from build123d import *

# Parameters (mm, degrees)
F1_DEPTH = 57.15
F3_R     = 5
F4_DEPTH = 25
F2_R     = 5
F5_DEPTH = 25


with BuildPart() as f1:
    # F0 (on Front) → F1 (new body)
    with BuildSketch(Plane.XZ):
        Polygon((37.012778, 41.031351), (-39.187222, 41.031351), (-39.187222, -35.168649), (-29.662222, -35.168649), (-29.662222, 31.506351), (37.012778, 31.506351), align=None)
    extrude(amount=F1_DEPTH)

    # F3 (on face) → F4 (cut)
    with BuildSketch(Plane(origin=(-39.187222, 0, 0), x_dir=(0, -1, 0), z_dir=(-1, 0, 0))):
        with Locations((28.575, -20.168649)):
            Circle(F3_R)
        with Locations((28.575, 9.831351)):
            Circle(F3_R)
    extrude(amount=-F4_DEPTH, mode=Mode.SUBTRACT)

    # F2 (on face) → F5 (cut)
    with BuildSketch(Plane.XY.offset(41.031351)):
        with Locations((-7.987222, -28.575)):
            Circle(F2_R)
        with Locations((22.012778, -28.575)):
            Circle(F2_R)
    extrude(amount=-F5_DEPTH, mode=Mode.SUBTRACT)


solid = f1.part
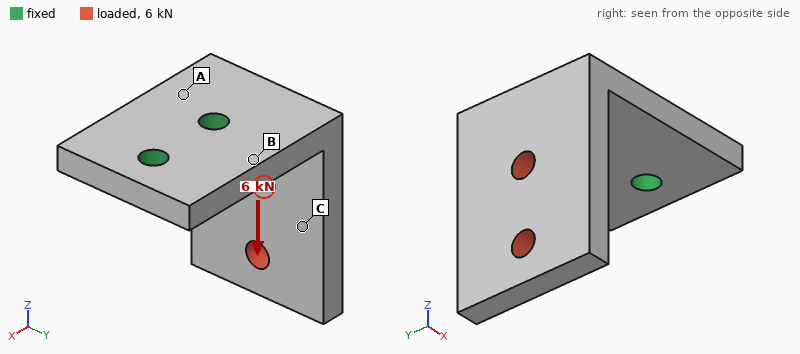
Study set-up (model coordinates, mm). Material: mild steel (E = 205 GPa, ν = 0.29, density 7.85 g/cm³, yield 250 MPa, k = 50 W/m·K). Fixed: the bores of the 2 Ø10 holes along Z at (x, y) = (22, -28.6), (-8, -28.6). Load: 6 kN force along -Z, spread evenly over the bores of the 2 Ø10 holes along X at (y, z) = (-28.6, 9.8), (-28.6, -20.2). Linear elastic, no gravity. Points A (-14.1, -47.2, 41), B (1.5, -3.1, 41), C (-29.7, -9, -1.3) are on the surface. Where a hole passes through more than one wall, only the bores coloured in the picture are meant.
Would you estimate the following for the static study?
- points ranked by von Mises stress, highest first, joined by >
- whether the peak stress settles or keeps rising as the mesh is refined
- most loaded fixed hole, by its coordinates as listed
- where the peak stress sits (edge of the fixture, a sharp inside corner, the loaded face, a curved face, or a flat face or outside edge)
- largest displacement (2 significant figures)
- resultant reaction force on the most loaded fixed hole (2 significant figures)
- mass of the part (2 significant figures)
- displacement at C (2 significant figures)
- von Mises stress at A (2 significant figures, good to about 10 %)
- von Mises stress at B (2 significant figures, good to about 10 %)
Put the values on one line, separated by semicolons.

A > B > C; keeps rising; (-8, -28.6); edge of the fixture; 0.19 mm; 7.5 kN; 590 g; 0.10 mm; 84 MPa; 41 MPa
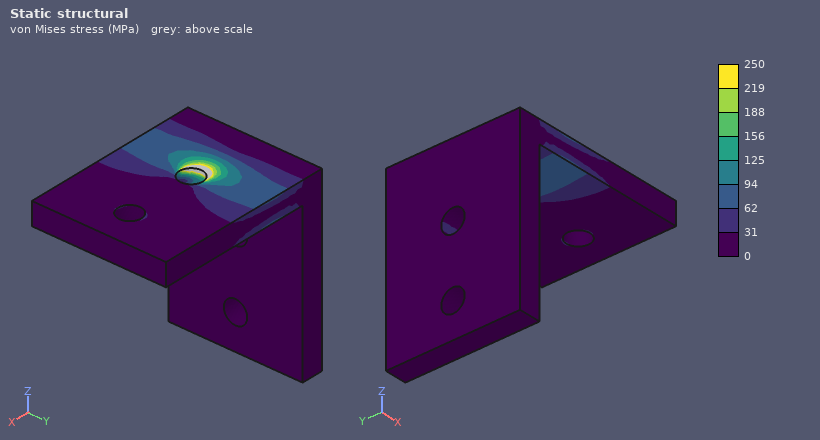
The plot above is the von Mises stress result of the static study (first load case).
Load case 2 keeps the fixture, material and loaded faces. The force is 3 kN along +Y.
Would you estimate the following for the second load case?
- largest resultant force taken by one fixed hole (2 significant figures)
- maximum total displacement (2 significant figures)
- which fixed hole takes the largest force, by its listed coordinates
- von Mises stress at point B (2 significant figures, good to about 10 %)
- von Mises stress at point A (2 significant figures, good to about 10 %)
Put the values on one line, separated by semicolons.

4.7 kN; 0.18 mm; (-8, -28.6); 52 MPa; 60 MPa
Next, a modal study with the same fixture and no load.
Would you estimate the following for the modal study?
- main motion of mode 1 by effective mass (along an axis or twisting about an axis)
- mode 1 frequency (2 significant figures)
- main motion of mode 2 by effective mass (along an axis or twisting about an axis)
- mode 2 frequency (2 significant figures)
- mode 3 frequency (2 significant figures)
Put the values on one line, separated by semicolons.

along X; 1000 Hz; along Y; 1500 Hz; 3700 Hz
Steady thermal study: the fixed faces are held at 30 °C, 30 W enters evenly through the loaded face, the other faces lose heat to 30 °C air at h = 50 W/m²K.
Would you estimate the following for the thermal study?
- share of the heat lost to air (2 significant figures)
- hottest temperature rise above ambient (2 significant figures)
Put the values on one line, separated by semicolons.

55 %; 44 K
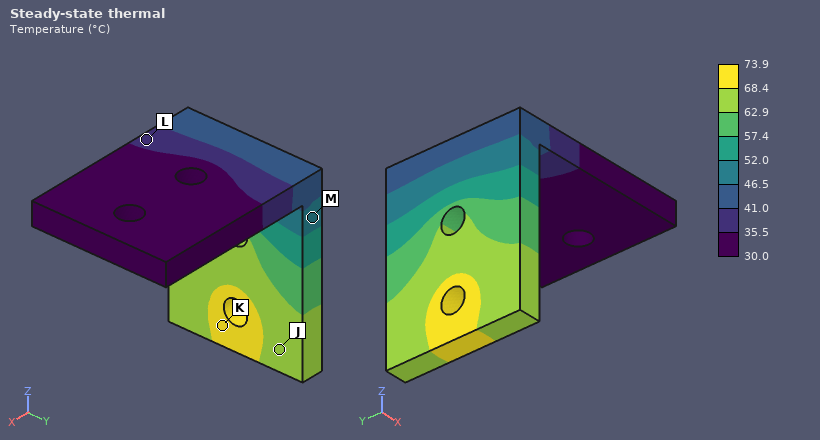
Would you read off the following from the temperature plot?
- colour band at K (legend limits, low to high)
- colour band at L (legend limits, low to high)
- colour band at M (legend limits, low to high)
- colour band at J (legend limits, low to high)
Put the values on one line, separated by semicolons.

68.4 to 73.9 °C; 35.5 to 41.0 °C; 46.5 to 52.0 °C; 62.9 to 68.4 °C
